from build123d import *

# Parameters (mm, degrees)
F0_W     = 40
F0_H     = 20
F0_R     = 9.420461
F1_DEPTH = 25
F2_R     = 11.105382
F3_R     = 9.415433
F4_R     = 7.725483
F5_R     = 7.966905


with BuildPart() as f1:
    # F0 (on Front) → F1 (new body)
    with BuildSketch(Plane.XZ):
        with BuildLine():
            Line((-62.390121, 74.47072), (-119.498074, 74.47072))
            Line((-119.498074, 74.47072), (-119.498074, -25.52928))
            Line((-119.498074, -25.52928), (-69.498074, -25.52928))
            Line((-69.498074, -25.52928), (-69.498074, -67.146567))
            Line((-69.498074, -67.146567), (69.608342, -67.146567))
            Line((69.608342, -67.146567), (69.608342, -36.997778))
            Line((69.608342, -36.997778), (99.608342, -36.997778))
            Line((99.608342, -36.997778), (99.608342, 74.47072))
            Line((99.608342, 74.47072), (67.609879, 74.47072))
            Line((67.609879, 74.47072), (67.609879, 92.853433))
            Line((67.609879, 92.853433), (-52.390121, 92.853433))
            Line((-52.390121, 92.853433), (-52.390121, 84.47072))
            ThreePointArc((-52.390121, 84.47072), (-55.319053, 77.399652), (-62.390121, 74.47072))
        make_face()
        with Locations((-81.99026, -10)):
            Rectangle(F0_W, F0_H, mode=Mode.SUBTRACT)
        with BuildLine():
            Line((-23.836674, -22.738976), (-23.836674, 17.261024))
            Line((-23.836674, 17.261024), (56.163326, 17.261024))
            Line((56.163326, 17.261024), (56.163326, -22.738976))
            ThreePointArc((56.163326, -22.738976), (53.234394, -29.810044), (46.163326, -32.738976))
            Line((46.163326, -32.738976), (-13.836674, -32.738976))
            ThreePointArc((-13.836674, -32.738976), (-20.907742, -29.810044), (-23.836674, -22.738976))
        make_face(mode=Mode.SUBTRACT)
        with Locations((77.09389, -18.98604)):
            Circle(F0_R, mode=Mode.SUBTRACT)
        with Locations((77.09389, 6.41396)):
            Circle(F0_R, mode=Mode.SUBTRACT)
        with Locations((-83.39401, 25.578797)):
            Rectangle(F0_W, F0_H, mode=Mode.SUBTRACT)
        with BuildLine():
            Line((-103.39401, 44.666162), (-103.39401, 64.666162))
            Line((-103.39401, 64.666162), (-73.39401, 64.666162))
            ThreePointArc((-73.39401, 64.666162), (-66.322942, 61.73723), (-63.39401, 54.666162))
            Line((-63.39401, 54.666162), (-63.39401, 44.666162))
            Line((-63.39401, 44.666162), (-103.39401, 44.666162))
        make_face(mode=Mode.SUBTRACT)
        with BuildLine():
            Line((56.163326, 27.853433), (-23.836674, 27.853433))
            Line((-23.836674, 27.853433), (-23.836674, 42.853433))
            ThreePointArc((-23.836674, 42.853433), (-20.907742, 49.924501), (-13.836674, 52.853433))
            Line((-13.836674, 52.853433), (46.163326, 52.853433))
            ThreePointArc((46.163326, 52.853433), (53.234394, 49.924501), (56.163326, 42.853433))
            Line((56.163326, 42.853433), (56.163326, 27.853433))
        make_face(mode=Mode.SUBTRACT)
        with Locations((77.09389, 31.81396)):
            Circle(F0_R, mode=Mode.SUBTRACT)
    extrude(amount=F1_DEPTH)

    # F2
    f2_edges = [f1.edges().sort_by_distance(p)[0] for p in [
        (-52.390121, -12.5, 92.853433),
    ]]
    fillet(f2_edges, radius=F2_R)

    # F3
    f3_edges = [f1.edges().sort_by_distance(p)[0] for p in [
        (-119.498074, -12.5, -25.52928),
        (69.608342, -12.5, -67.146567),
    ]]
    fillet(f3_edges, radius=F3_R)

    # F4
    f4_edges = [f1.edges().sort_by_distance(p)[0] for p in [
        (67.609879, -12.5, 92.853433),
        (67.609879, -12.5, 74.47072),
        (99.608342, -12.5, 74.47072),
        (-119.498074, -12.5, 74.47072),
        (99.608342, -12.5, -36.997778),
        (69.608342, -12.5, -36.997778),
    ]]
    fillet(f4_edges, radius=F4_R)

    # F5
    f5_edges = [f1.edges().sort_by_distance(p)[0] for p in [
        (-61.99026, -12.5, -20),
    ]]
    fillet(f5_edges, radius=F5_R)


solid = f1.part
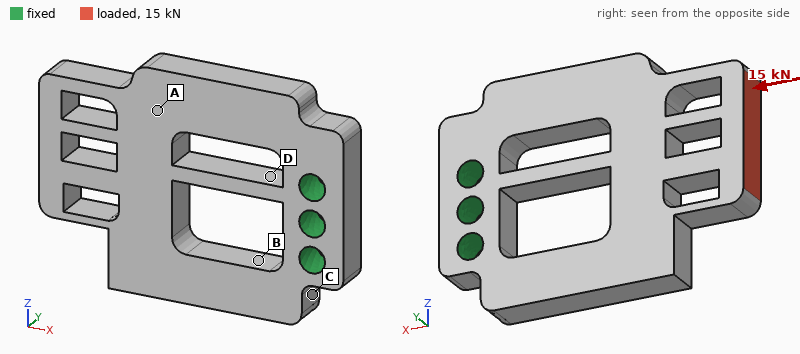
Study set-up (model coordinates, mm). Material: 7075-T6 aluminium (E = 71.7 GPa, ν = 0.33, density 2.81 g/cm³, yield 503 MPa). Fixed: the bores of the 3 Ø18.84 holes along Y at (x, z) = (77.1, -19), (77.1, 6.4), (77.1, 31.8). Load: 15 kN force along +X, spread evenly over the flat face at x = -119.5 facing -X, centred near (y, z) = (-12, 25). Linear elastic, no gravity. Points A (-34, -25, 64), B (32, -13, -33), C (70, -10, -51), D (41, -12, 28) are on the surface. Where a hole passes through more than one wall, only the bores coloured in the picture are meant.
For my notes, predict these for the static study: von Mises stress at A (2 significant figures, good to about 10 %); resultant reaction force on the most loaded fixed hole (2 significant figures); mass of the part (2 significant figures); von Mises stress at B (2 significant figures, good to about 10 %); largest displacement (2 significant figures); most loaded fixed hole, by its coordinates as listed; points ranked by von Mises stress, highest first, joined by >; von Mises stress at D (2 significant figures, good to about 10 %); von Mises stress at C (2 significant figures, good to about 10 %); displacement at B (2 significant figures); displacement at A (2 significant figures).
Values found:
8.3 MPa
11 kN
1.5 kg
12 MPa
50 µm
(77.1, 31.8)
D > B > A > C
24 MPa
2.9 MPa
9.1 µm
30 µm
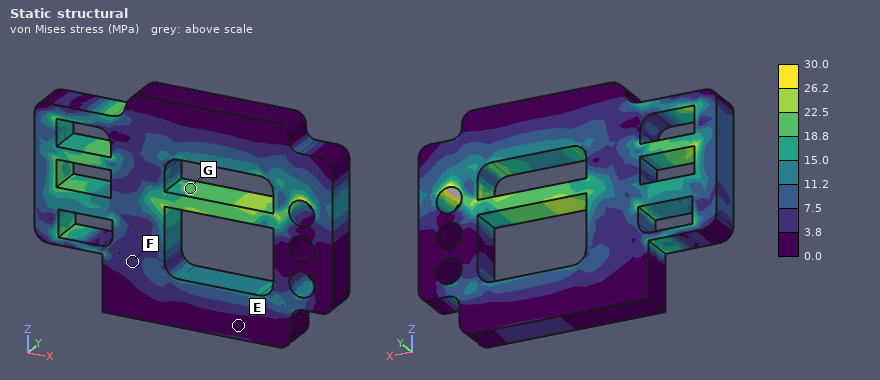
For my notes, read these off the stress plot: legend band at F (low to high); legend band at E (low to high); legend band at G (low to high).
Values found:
3.8 to 7.5 MPa
0.0 to 3.8 MPa
18.8 to 22.5 MPa
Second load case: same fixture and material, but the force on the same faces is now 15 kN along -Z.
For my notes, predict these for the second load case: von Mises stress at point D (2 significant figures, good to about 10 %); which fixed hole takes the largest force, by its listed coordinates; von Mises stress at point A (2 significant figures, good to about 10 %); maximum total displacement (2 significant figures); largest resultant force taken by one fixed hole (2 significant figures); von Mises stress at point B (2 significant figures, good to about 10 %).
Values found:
76 MPa
(77.1, 31.8)
22 MPa
0.94 mm
34 kN
50 MPa
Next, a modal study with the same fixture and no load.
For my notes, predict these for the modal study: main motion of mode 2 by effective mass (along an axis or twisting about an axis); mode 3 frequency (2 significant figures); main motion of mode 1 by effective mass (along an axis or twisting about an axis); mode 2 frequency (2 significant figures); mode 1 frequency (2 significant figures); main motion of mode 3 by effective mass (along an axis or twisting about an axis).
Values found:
along Z
1200 Hz
along Y
960 Hz
470 Hz
twisting about X
